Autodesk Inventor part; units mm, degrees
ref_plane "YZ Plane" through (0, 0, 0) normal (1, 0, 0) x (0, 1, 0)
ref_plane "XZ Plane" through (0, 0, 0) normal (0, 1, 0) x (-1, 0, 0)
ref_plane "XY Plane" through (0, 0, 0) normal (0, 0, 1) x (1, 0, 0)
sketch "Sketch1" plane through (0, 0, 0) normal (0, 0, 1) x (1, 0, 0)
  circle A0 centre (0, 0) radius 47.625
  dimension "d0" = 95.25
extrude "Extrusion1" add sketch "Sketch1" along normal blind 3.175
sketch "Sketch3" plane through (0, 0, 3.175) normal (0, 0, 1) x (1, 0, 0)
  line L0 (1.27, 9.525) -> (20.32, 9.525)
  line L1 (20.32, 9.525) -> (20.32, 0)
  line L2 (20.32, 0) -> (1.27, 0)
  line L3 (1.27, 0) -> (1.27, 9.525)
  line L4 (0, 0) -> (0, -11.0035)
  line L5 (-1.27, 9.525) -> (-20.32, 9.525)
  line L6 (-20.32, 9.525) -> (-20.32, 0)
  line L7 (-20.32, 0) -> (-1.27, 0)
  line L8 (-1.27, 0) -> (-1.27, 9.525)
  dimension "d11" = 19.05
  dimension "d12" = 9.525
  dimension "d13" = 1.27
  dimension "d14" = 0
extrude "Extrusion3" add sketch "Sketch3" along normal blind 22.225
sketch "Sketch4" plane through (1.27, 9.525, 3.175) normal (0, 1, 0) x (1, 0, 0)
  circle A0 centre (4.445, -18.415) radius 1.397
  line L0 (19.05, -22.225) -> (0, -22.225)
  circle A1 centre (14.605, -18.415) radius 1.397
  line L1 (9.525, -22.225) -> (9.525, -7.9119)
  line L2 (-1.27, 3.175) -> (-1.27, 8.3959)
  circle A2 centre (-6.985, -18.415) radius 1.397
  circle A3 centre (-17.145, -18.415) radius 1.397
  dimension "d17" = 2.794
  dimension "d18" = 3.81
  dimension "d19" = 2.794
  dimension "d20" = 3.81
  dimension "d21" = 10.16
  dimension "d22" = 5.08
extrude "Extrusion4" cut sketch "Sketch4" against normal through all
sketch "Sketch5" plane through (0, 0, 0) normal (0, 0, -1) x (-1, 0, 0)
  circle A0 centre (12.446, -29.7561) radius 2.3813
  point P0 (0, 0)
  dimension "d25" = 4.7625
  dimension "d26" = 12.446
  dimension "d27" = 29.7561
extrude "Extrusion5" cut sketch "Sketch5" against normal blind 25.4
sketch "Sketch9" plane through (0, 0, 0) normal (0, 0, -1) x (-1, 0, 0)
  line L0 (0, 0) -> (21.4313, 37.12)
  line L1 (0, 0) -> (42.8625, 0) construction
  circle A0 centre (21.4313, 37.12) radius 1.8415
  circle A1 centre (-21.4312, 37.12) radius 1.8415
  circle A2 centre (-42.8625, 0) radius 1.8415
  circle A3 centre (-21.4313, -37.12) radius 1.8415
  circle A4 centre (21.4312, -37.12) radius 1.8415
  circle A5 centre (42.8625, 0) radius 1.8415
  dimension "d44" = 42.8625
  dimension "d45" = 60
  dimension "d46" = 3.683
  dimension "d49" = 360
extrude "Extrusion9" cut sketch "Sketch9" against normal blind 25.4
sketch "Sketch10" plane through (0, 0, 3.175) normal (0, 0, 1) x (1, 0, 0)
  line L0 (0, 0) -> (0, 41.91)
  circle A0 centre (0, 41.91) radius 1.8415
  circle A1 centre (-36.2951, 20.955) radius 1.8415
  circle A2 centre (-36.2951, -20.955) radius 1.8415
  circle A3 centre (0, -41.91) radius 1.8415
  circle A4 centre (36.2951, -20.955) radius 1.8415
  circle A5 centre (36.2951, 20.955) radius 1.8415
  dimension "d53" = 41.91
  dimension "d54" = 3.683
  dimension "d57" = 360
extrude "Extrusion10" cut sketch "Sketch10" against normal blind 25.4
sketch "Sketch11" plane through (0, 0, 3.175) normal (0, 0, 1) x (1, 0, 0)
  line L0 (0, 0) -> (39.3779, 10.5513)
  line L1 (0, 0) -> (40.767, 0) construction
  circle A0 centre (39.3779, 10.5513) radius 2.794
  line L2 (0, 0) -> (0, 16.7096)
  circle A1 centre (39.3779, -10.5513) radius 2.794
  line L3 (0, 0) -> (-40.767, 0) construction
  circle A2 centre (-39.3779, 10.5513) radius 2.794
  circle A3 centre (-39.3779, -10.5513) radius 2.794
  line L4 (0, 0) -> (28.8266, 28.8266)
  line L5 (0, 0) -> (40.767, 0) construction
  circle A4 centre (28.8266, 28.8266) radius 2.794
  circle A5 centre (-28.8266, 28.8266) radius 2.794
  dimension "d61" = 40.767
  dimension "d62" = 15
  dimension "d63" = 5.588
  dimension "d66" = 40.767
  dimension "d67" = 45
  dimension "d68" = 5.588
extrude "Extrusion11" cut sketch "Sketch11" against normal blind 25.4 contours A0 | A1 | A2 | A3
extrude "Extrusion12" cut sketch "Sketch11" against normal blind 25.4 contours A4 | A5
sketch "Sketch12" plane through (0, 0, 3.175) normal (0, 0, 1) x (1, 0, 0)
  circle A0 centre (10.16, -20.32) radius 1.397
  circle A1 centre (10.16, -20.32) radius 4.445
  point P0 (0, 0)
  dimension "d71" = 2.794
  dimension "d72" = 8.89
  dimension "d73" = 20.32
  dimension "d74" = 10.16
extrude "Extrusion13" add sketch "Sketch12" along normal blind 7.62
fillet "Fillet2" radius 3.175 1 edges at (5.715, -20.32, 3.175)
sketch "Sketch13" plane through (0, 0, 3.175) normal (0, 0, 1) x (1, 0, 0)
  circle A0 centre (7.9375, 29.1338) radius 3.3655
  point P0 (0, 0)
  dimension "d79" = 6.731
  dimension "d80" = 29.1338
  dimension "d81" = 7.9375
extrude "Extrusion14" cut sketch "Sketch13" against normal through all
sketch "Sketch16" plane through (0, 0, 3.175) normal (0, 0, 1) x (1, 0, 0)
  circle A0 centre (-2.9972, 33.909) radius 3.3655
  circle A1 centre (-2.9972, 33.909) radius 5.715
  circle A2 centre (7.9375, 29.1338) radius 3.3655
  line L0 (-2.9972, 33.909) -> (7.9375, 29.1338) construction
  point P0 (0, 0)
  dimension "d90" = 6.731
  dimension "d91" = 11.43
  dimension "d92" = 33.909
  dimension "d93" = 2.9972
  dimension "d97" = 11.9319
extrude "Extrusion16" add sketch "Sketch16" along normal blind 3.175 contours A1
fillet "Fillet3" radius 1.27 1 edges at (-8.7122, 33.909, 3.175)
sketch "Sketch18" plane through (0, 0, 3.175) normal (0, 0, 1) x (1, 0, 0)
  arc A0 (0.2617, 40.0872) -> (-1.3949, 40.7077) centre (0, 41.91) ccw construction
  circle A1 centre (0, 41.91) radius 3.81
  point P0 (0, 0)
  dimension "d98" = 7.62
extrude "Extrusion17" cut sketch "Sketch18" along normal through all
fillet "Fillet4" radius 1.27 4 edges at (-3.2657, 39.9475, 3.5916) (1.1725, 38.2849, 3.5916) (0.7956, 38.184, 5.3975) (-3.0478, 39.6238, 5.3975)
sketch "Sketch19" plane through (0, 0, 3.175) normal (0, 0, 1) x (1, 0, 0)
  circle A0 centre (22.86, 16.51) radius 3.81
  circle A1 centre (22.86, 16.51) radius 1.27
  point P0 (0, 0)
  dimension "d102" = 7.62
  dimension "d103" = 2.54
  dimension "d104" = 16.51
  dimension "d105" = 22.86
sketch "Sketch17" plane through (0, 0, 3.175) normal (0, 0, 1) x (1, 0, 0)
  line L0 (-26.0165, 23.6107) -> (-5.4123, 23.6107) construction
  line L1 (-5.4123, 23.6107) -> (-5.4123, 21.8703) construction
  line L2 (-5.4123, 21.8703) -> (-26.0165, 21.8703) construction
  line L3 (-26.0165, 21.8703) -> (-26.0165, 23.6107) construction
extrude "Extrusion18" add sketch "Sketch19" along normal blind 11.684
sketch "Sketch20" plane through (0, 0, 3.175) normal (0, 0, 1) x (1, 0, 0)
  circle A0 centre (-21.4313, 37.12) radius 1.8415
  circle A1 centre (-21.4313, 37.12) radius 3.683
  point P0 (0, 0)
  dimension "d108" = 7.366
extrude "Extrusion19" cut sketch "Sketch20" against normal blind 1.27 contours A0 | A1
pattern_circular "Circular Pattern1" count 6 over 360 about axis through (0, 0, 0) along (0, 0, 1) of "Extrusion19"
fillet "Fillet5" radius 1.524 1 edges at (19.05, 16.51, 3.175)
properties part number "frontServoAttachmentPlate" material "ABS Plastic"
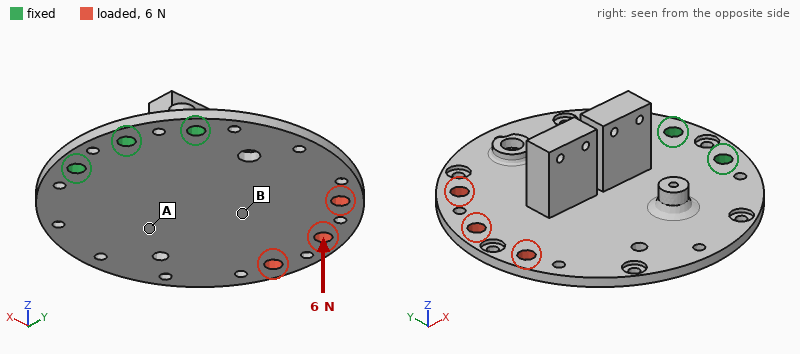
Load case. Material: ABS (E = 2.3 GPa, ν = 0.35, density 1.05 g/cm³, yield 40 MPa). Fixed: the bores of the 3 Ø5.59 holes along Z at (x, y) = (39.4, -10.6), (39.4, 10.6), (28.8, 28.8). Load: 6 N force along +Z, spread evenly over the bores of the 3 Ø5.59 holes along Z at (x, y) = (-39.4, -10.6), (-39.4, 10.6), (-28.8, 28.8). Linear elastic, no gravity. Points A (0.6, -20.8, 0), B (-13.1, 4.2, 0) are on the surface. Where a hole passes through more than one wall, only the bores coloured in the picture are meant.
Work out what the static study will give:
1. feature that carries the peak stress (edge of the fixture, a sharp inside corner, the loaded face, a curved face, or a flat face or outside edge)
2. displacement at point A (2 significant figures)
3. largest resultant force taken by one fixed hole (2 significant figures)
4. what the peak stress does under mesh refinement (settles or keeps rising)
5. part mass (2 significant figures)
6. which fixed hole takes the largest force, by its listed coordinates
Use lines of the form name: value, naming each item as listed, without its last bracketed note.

feature that carries the peak stress: edge of the fixture
displacement at point A: 0.42 mm
largest resultant force taken by one fixed hole: 8.5 N
what the peak stress does under mesh refinement: keeps rising
part mass: 32 g
which fixed hole takes the largest force, by its listed coordinates: (28.8, 28.8)
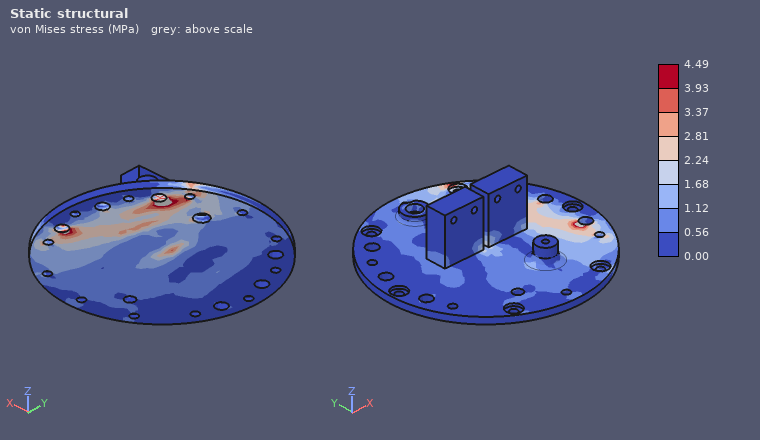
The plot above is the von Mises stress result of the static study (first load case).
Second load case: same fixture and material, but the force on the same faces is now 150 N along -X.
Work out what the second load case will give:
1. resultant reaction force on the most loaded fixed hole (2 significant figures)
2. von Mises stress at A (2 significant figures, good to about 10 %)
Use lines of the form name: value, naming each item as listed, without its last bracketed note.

resultant reaction force on the most loaded fixed hole: 57 N
von Mises stress at A: 0.45 MPa
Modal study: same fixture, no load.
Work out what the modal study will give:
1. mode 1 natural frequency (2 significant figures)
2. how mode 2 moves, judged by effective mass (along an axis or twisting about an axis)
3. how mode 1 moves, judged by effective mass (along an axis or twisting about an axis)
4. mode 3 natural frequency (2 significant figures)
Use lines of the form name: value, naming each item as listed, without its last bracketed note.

mode 1 natural frequency: 130 Hz
how mode 2 moves, judged by effective mass: twisting about X
how mode 1 moves, judged by effective mass: along Z
mode 3 natural frequency: 640 Hz
